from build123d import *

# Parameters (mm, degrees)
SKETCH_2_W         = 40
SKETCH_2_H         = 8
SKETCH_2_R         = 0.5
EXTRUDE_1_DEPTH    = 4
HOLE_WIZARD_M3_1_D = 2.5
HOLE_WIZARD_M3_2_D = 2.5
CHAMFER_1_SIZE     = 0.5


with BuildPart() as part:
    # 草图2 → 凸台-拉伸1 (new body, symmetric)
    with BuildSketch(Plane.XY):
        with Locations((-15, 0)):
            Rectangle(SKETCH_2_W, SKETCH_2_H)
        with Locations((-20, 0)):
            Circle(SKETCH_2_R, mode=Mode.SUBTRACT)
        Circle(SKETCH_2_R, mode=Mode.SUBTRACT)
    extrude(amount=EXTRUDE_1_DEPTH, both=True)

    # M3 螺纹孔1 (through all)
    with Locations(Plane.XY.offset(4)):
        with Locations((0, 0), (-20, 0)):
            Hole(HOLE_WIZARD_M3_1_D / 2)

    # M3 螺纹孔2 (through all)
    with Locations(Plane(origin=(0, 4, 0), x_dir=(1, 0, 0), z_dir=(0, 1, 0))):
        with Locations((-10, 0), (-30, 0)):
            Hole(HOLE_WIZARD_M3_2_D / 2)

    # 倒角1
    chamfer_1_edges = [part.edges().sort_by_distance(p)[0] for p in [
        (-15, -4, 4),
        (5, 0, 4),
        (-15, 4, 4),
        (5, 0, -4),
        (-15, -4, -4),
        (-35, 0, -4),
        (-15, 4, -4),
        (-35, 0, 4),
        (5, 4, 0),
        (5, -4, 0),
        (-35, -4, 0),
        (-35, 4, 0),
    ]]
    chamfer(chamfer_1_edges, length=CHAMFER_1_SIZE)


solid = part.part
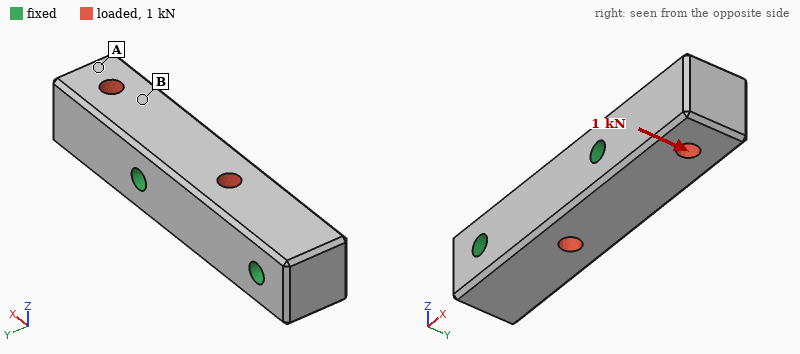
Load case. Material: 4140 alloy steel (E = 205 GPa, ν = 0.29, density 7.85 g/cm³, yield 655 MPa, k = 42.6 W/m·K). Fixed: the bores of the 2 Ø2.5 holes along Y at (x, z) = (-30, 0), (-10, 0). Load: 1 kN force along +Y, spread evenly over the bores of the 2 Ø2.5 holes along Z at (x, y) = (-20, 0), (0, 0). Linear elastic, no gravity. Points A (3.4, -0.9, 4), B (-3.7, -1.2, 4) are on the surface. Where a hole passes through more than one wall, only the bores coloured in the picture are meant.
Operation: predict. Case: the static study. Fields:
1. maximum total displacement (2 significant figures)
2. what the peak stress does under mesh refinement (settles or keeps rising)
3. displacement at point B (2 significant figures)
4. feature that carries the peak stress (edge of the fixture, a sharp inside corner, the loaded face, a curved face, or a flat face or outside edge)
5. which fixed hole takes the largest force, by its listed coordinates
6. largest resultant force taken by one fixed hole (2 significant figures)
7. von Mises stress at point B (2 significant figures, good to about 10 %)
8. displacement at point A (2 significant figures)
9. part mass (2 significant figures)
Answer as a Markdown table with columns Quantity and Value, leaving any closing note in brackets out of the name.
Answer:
| Quantity | Value |
|---|---|
| maximum total displacement | 5.6 µm |
| what the peak stress does under mesh refinement | keeps rising |
| displacement at point B | 1.7 µm |
| feature that carries the peak stress | edge of the fixture |
| which fixed hole takes the largest force, by its listed coordinates | (-10, 0) |
| largest resultant force taken by one fixed hole | 780 N |
| von Mises stress at point B | 21 MPa |
| displacement at point A | 4.9 µm |
| part mass | 19 g |
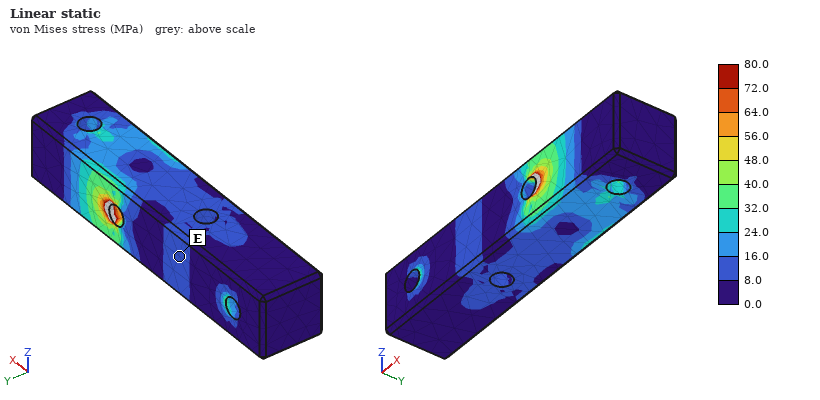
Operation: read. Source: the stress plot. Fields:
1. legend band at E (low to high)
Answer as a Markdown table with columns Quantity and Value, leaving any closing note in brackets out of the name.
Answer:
| Quantity | Value |
|---|---|
| legend band at E | 8.0 to 16.0 MPa |
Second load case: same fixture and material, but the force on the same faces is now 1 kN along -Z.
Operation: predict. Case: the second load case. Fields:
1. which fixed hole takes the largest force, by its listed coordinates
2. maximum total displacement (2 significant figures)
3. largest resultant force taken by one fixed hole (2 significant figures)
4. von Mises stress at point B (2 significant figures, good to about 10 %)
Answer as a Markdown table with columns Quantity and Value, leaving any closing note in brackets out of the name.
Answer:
| Quantity | Value |
|---|---|
| which fixed hole takes the largest force, by its listed coordinates | (-10, 0) |
| maximum total displacement | 7.6 µm |
| largest resultant force taken by one fixed hole | 860 N |
| von Mises stress at point B | 23 MPa |
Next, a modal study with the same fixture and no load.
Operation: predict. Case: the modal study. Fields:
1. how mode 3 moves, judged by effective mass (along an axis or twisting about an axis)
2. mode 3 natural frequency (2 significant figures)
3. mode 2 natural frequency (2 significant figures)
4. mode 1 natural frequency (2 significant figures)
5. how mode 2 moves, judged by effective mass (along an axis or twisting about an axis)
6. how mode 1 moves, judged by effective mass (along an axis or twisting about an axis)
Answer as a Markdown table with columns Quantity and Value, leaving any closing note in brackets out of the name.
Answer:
| Quantity | Value |
|---|---|
| how mode 3 moves, judged by effective mass | twisting about X |
| mode 3 natural frequency | 49 kHz |
| mode 2 natural frequency | 25 kHz |
| mode 1 natural frequency | 21 kHz |
| how mode 2 moves, judged by effective mass | along Y |
| how mode 1 moves, judged by effective mass | along Z |
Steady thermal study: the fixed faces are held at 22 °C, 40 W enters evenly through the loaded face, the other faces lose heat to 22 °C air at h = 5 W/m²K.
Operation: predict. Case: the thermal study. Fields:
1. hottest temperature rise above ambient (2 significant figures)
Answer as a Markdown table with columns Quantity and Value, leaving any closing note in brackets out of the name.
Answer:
| Quantity | Value |
|---|---|
| hottest temperature rise above ambient | 84 K |
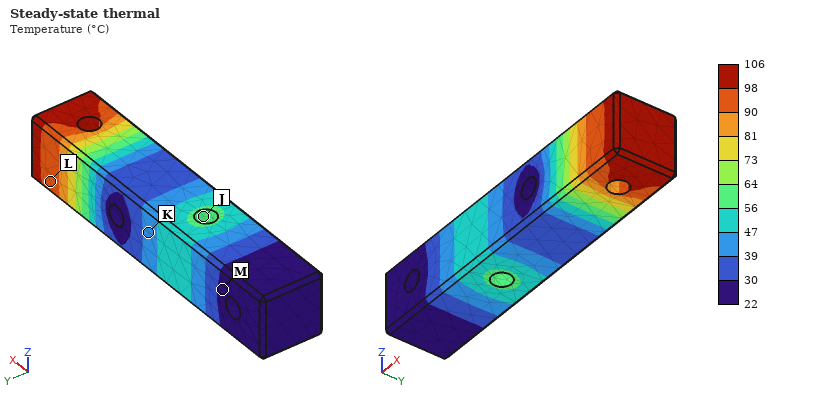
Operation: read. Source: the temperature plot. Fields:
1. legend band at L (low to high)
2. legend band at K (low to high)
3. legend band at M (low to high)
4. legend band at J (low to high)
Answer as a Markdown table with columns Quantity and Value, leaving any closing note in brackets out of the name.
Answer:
| Quantity | Value |
|---|---|
| legend band at L | 90 to 98 °C |
| legend band at K | 39 to 47 °C |
| legend band at M | 22 to 30 °C |
| legend band at J | 56 to 64 °C |
